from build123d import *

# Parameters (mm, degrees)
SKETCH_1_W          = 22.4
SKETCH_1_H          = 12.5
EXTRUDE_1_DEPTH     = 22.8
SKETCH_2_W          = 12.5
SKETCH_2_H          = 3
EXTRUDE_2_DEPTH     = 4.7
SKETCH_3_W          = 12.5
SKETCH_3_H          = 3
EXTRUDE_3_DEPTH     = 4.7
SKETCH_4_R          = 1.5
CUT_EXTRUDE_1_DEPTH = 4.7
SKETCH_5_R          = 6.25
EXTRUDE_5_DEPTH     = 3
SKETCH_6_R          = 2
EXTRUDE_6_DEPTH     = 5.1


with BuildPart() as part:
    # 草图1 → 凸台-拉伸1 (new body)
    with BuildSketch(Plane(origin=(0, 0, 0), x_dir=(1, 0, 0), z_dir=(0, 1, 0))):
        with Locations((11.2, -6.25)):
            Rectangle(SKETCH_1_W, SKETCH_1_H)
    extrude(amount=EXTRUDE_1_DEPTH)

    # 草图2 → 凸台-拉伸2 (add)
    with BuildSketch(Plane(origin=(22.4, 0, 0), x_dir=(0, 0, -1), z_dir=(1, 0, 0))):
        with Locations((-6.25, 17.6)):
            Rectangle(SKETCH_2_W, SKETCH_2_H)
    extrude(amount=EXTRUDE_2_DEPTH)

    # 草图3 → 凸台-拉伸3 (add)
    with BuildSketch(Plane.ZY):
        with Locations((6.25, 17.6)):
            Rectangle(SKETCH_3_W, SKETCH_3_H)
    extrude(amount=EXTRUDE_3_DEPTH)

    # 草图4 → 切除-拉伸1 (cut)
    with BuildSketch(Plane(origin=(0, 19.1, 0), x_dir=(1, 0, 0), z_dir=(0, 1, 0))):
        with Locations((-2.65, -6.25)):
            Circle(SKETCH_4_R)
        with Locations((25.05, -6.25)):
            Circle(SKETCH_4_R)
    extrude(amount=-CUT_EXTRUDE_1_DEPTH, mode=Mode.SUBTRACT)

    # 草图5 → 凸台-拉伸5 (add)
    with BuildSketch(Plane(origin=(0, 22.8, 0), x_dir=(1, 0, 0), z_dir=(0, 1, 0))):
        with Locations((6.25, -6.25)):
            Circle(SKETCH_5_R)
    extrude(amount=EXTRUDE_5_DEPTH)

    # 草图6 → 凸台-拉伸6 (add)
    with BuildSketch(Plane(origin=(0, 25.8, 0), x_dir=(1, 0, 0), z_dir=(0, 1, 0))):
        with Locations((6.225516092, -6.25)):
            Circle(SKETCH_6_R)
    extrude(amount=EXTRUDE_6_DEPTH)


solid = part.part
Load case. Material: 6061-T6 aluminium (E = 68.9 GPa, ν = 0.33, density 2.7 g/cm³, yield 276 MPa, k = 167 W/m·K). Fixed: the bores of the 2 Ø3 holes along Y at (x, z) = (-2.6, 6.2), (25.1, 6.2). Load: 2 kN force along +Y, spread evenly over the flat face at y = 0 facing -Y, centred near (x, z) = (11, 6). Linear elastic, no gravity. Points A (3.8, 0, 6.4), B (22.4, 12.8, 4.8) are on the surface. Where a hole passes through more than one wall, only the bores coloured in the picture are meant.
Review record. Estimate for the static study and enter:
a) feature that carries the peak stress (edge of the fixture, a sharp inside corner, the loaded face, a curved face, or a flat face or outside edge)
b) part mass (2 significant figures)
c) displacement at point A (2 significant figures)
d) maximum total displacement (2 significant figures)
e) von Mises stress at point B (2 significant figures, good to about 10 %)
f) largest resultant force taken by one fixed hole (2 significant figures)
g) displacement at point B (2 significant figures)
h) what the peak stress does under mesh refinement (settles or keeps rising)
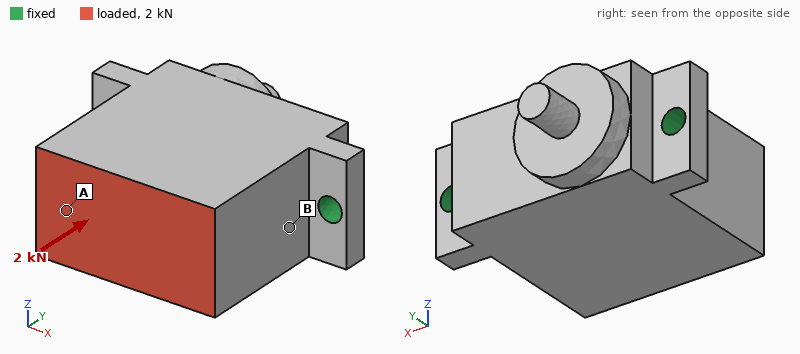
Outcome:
edge of the fixture
19 g
8.9 µm
9.1 µm
24 MPa
1.0 kN
7.2 µm
keeps rising
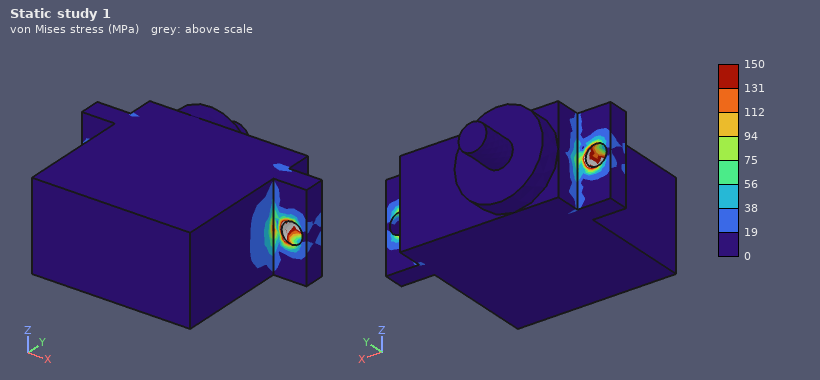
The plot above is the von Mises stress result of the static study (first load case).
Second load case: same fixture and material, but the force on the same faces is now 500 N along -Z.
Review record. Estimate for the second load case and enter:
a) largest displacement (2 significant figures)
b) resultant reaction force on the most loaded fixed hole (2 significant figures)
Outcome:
87 µm
250 N
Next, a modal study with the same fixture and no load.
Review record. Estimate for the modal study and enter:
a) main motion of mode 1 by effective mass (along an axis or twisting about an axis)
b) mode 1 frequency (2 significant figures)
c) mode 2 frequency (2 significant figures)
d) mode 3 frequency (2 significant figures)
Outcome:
along Z
5300 Hz
19 kHz
19 kHz
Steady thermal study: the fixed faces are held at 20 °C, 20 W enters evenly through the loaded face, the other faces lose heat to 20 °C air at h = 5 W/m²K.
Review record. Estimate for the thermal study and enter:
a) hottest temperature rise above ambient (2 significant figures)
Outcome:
15 K
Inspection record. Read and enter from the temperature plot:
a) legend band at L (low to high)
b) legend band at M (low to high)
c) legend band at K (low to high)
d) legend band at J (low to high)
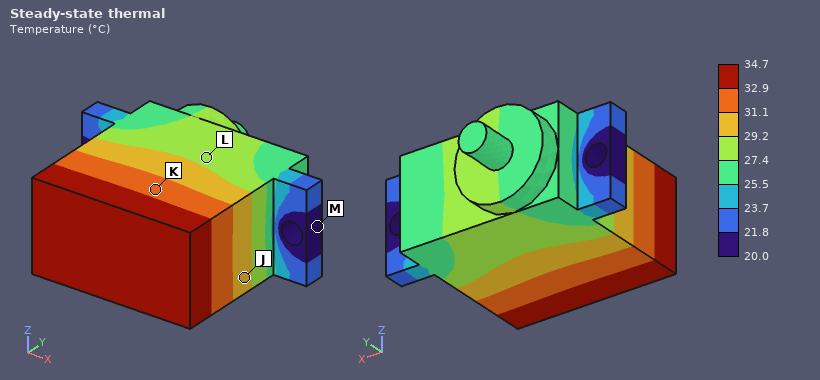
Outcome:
27.4 to 29.2 °C
20.0 to 21.8 °C
31.1 to 32.9 °C
29.2 to 31.1 °C
